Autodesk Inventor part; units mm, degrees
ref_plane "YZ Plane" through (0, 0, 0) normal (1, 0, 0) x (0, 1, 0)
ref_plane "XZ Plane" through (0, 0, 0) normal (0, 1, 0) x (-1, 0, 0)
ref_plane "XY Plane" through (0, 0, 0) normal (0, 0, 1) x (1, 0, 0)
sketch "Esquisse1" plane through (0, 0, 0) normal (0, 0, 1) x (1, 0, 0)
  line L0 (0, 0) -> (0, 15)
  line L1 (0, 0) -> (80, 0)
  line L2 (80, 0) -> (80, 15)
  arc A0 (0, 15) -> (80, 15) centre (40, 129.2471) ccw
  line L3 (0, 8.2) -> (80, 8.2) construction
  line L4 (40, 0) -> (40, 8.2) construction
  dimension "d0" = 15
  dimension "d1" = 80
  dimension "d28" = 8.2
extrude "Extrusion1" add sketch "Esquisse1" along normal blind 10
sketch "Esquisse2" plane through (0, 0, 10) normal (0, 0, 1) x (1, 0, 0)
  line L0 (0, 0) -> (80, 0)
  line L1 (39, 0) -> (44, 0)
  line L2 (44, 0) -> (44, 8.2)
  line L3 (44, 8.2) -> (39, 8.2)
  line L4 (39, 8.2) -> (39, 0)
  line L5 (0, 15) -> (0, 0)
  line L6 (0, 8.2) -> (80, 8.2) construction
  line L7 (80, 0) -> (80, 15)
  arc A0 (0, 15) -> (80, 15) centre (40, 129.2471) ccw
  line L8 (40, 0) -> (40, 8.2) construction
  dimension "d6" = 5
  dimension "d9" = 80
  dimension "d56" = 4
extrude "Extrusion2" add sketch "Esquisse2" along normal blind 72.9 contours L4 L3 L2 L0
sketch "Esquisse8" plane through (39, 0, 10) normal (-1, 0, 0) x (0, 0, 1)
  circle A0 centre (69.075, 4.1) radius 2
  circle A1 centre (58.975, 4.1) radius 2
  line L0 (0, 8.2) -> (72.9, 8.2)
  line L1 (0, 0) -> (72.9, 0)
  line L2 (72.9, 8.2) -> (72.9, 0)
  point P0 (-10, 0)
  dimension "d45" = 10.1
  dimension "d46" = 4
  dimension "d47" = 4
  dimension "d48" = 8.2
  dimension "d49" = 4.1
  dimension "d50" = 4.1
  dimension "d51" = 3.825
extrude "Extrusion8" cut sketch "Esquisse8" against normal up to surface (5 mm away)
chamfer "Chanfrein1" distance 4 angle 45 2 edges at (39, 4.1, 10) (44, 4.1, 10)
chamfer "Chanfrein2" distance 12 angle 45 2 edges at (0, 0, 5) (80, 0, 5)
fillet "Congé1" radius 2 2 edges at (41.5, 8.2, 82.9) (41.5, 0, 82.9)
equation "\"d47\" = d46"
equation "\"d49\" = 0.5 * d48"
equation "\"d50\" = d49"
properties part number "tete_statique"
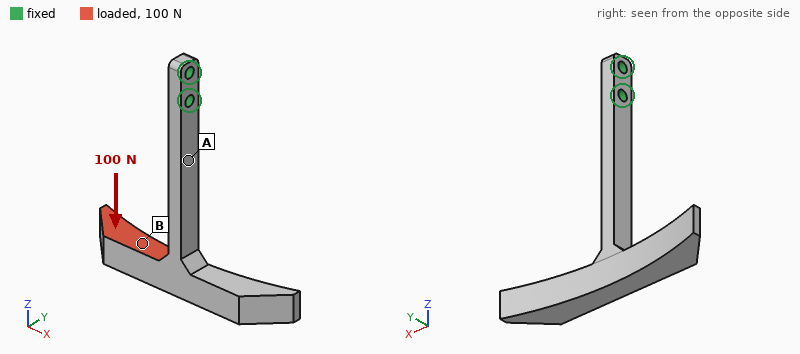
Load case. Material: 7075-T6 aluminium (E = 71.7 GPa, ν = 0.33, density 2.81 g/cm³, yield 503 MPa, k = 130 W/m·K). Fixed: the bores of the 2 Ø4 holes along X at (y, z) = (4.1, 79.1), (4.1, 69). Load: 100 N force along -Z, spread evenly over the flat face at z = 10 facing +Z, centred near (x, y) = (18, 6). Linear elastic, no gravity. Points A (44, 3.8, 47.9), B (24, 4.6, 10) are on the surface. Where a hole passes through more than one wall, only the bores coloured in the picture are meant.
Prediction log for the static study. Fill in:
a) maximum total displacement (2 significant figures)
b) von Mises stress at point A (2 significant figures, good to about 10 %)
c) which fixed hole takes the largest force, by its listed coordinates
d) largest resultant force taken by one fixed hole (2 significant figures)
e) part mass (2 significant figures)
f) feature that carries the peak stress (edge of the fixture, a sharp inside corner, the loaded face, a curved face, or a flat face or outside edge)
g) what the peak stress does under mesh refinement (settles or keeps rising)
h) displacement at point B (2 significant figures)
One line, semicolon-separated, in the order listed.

1.2 mm; 65 MPa; (4.1, 69); 97 N; 28 g; edge of the fixture; keeps rising; 0.73 mm
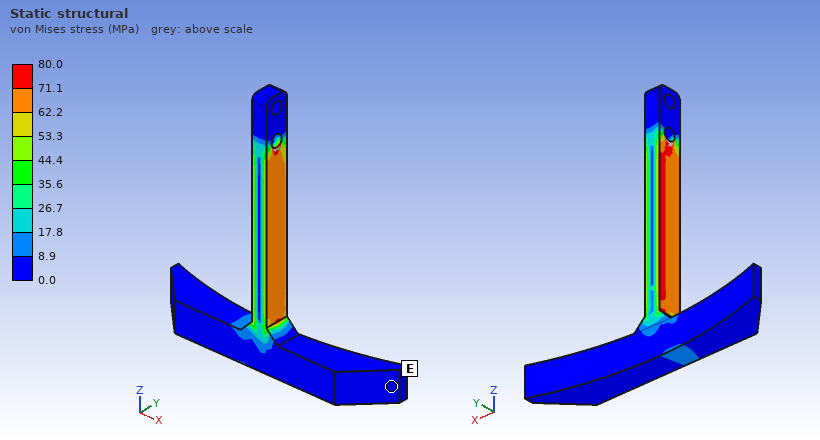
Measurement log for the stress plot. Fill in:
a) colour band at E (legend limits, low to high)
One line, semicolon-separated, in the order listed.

0.0 to 8.9 MPa
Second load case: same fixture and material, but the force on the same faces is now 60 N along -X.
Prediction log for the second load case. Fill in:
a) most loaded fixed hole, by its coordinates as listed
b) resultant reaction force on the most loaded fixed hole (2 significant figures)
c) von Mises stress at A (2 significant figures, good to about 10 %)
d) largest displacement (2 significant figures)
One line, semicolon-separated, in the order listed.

(4.1, 69); 81 N; 67 MPa; 1.1 mm
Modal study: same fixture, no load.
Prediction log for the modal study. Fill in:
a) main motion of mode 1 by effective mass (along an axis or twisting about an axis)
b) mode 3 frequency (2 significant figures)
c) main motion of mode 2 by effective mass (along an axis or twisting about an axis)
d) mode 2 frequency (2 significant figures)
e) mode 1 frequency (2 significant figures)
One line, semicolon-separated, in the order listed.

along X; 530 Hz; along Y; 460 Hz; 270 Hz
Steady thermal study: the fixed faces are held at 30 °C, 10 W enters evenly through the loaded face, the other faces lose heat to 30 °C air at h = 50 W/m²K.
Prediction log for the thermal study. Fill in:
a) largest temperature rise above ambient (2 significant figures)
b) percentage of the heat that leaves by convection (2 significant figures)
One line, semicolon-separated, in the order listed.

52 K; 69 %
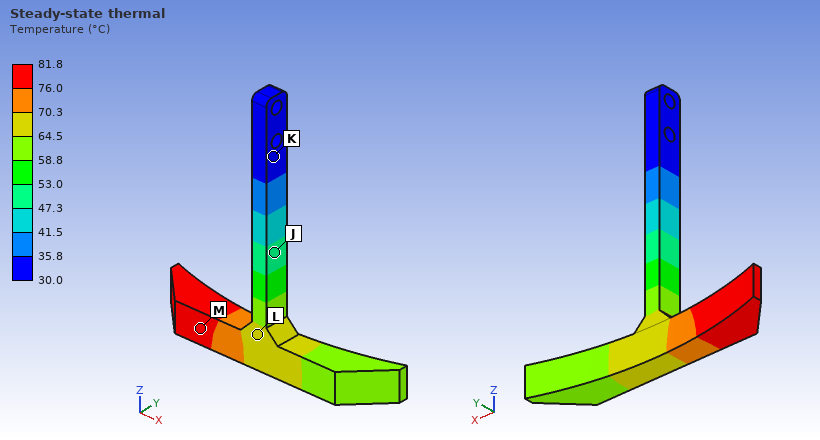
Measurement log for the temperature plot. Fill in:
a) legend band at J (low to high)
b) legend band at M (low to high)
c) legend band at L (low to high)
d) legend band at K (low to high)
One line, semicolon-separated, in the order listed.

47.3 to 53.0 °C; 76.0 to 81.8 °C; 64.5 to 70.3 °C; 30.0 to 35.8 °C
